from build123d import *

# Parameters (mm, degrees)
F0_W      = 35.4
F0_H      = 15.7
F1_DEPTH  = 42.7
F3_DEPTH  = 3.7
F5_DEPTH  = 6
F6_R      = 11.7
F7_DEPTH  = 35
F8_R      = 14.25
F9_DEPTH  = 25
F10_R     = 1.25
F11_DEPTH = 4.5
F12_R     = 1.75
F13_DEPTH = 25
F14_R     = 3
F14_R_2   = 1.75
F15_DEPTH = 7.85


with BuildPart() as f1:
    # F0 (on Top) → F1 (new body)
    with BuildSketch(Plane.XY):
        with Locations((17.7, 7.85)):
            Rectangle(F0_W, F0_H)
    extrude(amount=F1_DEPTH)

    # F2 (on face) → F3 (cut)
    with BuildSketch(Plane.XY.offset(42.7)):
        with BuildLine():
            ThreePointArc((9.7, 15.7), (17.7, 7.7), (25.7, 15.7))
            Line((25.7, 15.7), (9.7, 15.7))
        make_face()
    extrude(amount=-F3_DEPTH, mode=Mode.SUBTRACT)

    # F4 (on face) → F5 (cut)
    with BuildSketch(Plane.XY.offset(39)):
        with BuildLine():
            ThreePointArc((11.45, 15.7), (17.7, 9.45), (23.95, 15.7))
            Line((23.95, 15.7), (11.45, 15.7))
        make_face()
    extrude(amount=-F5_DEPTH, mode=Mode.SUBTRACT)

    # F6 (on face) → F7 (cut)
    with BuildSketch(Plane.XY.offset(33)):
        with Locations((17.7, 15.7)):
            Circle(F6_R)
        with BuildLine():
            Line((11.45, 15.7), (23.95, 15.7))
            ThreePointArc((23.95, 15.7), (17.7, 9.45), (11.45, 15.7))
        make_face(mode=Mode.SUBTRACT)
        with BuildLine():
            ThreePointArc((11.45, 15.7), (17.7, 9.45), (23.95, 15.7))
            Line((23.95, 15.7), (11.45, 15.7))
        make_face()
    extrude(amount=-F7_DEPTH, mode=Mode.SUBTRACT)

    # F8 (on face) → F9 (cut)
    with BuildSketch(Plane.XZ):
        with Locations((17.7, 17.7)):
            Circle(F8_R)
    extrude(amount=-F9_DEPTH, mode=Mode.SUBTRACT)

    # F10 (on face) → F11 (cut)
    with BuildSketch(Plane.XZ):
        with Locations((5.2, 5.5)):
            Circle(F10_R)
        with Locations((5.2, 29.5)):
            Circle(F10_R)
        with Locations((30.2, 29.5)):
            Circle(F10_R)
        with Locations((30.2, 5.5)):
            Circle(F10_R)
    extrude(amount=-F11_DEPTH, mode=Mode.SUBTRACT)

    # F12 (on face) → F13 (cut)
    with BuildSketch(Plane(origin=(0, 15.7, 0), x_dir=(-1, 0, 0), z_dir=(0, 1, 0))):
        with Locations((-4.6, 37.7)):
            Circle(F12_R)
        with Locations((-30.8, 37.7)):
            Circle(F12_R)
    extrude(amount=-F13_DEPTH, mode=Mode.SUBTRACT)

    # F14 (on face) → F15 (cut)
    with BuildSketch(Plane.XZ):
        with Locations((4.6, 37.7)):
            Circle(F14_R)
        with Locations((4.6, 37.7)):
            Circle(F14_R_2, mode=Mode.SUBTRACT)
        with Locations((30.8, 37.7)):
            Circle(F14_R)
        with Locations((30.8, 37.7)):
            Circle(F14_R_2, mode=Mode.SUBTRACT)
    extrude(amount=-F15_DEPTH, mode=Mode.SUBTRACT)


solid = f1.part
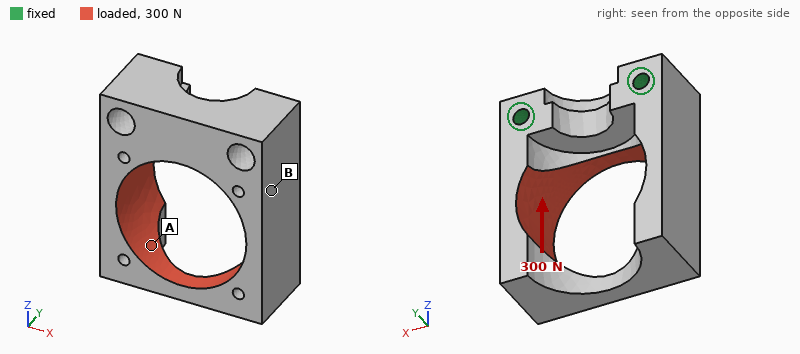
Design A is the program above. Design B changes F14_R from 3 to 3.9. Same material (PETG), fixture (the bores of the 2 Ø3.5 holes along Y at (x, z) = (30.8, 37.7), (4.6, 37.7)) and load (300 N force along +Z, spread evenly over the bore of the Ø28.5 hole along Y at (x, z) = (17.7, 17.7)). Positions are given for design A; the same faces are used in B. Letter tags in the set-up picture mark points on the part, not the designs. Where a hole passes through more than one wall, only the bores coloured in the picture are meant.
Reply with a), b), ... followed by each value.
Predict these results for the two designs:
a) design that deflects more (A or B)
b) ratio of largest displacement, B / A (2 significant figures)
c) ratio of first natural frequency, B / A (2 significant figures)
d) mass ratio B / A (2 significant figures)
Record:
a) B
b) 1.1
c) 0.97
d) 0.97
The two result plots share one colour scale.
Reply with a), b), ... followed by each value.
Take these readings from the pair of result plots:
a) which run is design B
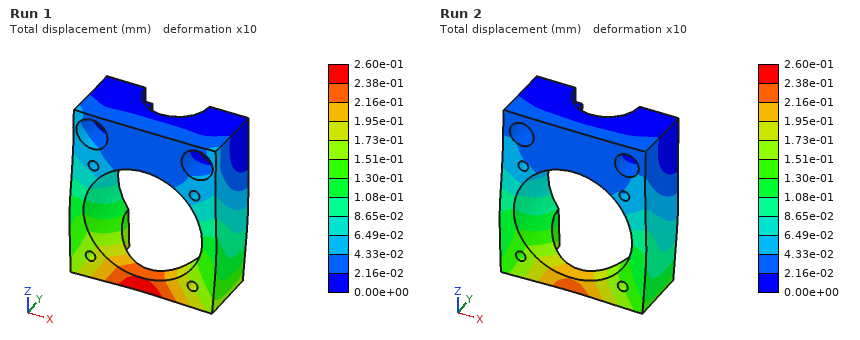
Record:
a) Run 1
